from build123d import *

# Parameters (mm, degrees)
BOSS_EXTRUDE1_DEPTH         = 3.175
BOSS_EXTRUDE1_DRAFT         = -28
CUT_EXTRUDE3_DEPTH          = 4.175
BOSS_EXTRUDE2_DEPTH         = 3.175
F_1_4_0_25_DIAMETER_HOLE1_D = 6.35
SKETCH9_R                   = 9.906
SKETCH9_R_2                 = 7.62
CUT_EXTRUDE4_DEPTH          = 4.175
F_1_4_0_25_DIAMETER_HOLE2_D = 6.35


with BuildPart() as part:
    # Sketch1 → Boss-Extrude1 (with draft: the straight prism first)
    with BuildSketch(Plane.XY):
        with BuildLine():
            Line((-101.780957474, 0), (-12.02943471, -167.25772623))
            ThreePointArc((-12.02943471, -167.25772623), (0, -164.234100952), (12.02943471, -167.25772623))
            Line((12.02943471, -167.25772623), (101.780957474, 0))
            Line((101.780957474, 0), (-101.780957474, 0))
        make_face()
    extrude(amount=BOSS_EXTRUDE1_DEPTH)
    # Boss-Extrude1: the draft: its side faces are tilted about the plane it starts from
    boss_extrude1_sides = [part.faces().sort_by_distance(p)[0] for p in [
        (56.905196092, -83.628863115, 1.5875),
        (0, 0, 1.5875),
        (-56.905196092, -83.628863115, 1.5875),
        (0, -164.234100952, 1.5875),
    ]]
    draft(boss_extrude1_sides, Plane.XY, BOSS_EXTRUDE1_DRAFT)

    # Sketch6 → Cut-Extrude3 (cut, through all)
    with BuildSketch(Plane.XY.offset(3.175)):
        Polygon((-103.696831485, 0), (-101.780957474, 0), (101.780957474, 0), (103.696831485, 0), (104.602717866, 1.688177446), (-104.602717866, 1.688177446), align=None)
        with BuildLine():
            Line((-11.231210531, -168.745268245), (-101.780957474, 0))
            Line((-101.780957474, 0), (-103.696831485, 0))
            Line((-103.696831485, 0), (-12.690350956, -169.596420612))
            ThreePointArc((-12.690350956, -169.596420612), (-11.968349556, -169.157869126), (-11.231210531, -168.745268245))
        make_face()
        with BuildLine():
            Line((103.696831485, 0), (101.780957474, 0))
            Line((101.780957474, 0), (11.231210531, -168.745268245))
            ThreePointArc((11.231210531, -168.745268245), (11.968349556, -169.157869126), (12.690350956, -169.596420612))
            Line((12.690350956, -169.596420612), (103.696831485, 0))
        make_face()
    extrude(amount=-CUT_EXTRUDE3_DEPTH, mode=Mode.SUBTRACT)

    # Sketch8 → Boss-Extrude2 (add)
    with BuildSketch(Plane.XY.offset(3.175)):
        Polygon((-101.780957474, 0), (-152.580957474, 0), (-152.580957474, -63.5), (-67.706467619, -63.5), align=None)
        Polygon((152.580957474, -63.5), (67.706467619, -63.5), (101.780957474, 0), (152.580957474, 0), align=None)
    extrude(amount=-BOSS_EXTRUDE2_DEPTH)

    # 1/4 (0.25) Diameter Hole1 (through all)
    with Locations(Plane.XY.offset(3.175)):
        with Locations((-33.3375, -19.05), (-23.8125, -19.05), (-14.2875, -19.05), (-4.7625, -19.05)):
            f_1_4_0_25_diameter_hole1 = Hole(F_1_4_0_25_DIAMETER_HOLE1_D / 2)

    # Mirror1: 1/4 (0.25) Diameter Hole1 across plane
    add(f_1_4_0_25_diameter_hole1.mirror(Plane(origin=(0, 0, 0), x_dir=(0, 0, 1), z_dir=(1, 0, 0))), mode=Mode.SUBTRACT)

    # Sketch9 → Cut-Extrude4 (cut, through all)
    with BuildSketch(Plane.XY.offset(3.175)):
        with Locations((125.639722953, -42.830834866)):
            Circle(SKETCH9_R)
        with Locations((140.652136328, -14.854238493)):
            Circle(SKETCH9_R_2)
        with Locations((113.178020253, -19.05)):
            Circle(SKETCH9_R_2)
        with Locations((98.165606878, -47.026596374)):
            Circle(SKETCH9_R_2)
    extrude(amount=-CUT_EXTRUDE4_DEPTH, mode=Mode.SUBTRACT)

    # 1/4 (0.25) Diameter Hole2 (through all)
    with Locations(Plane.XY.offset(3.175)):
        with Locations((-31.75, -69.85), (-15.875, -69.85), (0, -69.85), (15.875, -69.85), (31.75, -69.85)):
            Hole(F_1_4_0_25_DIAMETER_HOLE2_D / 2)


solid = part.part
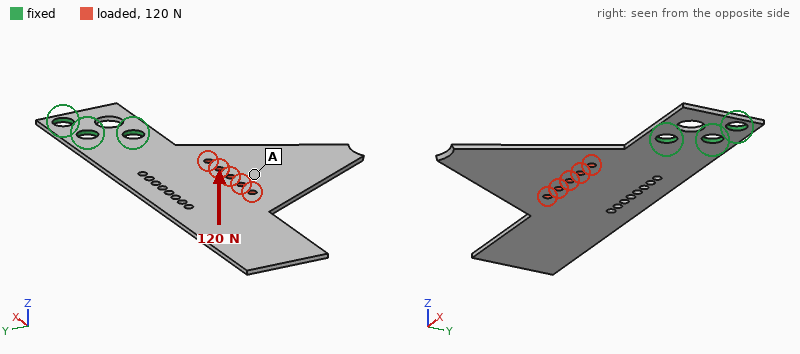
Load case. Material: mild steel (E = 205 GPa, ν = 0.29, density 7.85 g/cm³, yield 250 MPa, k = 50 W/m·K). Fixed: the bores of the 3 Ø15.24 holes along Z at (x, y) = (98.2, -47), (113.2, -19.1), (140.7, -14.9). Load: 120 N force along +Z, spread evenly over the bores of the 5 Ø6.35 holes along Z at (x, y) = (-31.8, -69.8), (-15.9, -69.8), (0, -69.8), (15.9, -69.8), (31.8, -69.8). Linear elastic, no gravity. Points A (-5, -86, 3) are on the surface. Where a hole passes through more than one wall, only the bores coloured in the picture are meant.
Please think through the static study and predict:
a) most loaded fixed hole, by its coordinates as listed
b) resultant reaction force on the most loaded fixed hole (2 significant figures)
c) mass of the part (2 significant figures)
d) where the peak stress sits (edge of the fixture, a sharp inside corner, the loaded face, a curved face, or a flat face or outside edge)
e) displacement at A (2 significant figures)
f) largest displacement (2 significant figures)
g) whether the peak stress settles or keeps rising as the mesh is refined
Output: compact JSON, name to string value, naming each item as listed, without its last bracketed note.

{"most loaded fixed hole, by its coordinates as listed": "(98.2, -47)", "resultant reaction force on the most loaded fixed hole": "260 N", "mass of the part": "660 g", "where the peak stress sits": "edge of the fixture", "displacement at A": "1.2 mm", "largest displacement": "3.2 mm", "whether the peak stress settles or keeps rising as the mesh is refined": "keeps rising"}
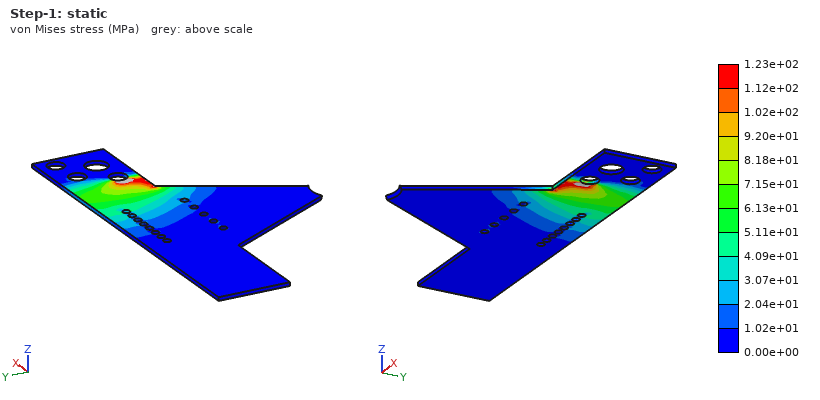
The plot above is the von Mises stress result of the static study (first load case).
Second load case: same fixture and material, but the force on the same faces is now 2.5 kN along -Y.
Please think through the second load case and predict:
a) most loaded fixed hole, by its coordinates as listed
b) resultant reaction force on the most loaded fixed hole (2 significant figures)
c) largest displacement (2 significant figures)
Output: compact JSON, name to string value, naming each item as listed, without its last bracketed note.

{"most loaded fixed hole, by its coordinates as listed": "(98.2, -47)", "resultant reaction force on the most loaded fixed hole": "6.3 kN", "largest displacement": "0.23 mm"}
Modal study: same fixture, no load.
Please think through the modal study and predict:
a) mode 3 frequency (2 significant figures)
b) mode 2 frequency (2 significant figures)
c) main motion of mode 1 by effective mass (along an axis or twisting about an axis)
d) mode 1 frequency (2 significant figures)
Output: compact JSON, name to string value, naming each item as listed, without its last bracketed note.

{"mode 3 frequency": "280 Hz", "mode 2 frequency": "130 Hz", "main motion of mode 1 by effective mass": "along Z", "mode 1 frequency": "44 Hz"}
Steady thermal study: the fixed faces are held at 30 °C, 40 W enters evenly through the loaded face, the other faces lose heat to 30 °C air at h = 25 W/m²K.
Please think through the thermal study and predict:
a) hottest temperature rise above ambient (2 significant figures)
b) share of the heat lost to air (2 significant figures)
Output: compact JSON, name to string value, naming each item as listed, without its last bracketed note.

{"hottest temperature rise above ambient": "75 K", "share of the heat lost to air": "89 %"}
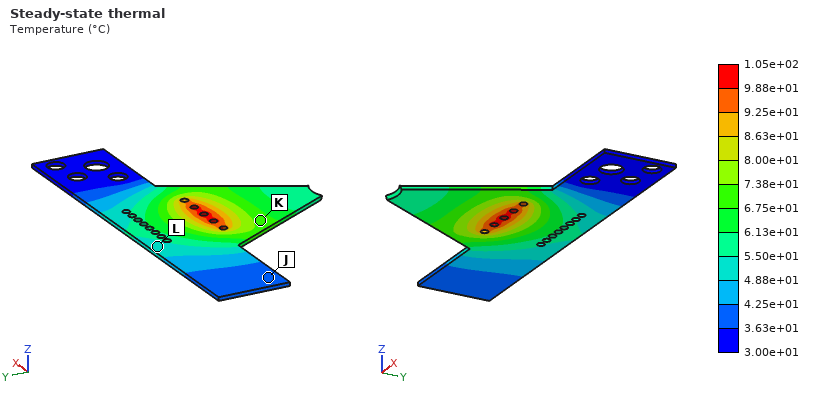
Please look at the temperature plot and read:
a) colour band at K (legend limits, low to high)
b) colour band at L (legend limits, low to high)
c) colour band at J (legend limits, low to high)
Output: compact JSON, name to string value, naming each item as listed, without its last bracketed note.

{"colour band at K": "6.75e+01 to 7.38e+01 °C", "colour band at L": "4.88e+01 to 5.50e+01 °C", "colour band at J": "3.63e+01 to 4.25e+01 °C"}
